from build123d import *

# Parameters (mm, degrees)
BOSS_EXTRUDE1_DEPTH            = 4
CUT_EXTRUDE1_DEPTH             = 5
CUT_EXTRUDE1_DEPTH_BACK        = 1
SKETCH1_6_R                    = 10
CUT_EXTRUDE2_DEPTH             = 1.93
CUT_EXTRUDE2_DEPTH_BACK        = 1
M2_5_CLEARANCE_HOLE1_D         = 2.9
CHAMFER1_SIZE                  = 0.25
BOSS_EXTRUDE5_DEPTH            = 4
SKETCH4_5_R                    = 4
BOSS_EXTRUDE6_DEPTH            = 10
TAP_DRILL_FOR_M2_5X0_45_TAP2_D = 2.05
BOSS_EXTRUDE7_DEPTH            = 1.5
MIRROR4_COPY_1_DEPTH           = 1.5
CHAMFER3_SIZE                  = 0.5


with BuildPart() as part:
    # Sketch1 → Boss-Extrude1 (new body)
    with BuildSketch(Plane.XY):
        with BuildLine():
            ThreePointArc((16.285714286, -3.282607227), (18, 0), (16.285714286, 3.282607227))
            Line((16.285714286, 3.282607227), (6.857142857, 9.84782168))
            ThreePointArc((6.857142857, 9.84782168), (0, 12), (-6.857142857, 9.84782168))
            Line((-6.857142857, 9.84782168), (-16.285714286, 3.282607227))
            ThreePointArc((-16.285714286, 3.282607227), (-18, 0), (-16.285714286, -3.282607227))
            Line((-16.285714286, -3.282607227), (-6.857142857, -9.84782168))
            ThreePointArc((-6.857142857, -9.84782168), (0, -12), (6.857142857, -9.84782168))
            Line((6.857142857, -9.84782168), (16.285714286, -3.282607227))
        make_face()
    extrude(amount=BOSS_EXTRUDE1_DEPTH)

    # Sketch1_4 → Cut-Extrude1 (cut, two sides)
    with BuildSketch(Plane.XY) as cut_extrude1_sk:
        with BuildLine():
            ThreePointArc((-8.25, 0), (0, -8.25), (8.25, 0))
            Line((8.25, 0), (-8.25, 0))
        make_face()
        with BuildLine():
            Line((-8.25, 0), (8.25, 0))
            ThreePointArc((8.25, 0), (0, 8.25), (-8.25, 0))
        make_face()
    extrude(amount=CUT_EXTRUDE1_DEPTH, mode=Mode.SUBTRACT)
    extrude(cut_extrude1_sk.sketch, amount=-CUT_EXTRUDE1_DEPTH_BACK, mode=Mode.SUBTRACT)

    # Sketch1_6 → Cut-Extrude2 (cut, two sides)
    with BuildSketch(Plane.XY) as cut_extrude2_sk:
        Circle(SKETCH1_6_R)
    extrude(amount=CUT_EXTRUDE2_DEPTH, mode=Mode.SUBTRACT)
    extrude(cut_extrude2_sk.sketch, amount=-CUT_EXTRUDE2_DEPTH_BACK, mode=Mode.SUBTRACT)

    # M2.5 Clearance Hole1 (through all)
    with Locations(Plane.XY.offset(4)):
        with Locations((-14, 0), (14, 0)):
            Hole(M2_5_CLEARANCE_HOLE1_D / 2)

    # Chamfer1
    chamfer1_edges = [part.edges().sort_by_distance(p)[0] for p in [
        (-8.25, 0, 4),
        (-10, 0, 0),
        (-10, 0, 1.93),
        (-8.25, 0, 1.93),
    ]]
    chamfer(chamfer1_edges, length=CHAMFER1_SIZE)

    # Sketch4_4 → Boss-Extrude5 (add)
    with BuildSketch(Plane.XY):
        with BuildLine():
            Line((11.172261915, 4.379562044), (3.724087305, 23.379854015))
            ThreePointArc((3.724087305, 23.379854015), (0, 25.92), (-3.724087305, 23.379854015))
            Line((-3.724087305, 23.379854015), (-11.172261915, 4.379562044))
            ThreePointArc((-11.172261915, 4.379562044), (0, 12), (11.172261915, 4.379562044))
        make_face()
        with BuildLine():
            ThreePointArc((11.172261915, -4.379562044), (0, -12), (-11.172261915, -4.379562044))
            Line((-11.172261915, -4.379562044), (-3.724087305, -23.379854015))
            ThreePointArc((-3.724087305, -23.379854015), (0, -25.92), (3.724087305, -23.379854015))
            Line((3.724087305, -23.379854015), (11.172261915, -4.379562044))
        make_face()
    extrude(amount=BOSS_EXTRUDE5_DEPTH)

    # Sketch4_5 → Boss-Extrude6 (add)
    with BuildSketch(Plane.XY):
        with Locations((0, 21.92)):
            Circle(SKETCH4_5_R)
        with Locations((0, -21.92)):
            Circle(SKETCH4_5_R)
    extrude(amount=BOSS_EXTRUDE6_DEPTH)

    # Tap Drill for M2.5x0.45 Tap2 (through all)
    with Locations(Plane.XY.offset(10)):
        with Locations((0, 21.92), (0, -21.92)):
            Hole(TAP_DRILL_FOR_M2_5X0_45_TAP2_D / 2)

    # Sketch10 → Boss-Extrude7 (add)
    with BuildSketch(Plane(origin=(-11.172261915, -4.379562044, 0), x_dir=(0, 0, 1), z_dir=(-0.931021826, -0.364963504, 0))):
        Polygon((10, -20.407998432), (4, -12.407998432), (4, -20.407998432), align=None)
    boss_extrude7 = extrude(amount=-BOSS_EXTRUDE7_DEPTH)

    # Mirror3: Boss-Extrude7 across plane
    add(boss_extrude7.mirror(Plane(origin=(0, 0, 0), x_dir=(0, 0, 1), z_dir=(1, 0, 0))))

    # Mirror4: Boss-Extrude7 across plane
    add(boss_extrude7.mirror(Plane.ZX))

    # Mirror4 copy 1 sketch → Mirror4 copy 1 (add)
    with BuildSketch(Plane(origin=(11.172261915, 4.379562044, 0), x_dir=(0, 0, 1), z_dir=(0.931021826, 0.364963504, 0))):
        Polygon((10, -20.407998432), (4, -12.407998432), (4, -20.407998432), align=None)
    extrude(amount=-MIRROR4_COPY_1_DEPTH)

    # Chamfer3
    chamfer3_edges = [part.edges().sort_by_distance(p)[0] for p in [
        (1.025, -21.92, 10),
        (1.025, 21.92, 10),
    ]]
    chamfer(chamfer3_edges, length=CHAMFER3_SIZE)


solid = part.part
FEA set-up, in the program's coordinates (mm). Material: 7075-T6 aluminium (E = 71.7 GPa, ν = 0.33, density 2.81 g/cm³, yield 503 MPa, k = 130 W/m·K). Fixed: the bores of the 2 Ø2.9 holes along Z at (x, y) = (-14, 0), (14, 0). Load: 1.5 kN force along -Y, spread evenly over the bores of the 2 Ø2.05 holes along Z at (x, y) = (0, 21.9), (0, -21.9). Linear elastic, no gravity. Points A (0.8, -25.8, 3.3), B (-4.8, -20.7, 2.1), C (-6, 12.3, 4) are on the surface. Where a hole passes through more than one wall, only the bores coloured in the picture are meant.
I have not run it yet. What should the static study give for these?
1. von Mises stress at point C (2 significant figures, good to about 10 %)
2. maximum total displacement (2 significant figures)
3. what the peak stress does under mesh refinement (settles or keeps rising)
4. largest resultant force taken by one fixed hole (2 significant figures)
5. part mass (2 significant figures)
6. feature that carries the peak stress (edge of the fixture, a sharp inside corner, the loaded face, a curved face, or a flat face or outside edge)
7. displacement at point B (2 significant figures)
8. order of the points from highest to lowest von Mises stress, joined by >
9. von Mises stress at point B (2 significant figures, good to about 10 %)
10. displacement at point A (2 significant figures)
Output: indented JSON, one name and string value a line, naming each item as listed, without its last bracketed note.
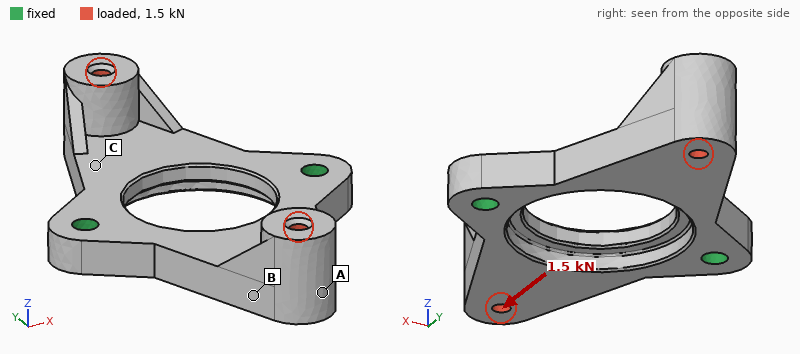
{
  "von Mises stress at point C": "81 MPa",
  "maximum total displacement": "0.23 mm",
  "what the peak stress does under mesh refinement": "keeps rising",
  "largest resultant force taken by one fixed hole": "750 N",
  "part mass": "8.9 g",
  "feature that carries the peak stress": "edge of the fixture",
  "displacement at point B": "0.14 mm",
  "order of the points from highest to lowest von Mises stress, joined by >": "C > B > A",
  "von Mises stress at point B": "32 MPa",
  "displacement at point A": "0.21 mm"
}
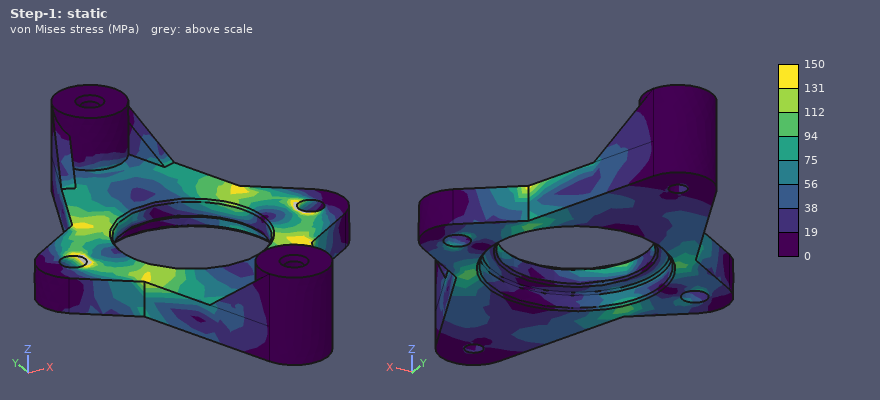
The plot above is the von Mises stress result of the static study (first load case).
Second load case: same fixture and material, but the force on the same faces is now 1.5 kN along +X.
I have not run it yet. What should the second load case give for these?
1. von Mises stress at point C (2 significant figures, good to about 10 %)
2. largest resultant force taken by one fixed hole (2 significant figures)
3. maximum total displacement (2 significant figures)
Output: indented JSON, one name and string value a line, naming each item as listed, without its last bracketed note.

{
  "von Mises stress at point C": "79 MPa",
  "largest resultant force taken by one fixed hole": "770 N",
  "maximum total displacement": "61 µm"
}
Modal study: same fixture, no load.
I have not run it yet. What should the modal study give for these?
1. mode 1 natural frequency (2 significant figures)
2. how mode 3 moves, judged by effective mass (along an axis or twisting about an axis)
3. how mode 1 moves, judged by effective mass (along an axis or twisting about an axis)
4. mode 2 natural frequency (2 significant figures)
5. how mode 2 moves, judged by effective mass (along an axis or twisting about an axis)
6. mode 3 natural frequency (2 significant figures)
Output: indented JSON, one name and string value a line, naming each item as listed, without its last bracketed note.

{
  "mode 1 natural frequency": "3100 Hz",
  "how mode 3 moves, judged by effective mass": "twisting about Z",
  "how mode 1 moves, judged by effective mass": "twisting about X",
  "mode 2 natural frequency": "3300 Hz",
  "how mode 2 moves, judged by effective mass": "along Z",
  "mode 3 natural frequency": "14 kHz"
}
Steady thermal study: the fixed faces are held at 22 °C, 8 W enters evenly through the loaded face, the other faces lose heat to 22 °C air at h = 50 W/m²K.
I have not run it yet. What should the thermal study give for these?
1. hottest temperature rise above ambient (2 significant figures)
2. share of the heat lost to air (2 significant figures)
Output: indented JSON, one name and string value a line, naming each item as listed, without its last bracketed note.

{
  "hottest temperature rise above ambient": "16 K",
  "share of the heat lost to air": "14 %"
}
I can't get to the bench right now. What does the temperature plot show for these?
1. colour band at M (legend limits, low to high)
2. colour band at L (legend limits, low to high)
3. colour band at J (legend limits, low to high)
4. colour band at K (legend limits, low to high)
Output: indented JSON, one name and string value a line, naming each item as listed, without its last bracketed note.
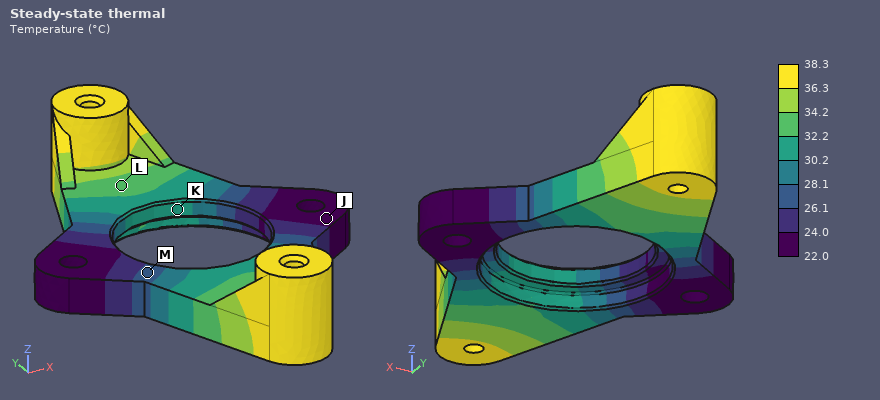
{
  "colour band at M": "26.1 to 28.1 °C",
  "colour band at L": "32.2 to 34.2 °C",
  "colour band at J": "22.0 to 24.0 °C",
  "colour band at K": "30.2 to 32.2 °C"
}
